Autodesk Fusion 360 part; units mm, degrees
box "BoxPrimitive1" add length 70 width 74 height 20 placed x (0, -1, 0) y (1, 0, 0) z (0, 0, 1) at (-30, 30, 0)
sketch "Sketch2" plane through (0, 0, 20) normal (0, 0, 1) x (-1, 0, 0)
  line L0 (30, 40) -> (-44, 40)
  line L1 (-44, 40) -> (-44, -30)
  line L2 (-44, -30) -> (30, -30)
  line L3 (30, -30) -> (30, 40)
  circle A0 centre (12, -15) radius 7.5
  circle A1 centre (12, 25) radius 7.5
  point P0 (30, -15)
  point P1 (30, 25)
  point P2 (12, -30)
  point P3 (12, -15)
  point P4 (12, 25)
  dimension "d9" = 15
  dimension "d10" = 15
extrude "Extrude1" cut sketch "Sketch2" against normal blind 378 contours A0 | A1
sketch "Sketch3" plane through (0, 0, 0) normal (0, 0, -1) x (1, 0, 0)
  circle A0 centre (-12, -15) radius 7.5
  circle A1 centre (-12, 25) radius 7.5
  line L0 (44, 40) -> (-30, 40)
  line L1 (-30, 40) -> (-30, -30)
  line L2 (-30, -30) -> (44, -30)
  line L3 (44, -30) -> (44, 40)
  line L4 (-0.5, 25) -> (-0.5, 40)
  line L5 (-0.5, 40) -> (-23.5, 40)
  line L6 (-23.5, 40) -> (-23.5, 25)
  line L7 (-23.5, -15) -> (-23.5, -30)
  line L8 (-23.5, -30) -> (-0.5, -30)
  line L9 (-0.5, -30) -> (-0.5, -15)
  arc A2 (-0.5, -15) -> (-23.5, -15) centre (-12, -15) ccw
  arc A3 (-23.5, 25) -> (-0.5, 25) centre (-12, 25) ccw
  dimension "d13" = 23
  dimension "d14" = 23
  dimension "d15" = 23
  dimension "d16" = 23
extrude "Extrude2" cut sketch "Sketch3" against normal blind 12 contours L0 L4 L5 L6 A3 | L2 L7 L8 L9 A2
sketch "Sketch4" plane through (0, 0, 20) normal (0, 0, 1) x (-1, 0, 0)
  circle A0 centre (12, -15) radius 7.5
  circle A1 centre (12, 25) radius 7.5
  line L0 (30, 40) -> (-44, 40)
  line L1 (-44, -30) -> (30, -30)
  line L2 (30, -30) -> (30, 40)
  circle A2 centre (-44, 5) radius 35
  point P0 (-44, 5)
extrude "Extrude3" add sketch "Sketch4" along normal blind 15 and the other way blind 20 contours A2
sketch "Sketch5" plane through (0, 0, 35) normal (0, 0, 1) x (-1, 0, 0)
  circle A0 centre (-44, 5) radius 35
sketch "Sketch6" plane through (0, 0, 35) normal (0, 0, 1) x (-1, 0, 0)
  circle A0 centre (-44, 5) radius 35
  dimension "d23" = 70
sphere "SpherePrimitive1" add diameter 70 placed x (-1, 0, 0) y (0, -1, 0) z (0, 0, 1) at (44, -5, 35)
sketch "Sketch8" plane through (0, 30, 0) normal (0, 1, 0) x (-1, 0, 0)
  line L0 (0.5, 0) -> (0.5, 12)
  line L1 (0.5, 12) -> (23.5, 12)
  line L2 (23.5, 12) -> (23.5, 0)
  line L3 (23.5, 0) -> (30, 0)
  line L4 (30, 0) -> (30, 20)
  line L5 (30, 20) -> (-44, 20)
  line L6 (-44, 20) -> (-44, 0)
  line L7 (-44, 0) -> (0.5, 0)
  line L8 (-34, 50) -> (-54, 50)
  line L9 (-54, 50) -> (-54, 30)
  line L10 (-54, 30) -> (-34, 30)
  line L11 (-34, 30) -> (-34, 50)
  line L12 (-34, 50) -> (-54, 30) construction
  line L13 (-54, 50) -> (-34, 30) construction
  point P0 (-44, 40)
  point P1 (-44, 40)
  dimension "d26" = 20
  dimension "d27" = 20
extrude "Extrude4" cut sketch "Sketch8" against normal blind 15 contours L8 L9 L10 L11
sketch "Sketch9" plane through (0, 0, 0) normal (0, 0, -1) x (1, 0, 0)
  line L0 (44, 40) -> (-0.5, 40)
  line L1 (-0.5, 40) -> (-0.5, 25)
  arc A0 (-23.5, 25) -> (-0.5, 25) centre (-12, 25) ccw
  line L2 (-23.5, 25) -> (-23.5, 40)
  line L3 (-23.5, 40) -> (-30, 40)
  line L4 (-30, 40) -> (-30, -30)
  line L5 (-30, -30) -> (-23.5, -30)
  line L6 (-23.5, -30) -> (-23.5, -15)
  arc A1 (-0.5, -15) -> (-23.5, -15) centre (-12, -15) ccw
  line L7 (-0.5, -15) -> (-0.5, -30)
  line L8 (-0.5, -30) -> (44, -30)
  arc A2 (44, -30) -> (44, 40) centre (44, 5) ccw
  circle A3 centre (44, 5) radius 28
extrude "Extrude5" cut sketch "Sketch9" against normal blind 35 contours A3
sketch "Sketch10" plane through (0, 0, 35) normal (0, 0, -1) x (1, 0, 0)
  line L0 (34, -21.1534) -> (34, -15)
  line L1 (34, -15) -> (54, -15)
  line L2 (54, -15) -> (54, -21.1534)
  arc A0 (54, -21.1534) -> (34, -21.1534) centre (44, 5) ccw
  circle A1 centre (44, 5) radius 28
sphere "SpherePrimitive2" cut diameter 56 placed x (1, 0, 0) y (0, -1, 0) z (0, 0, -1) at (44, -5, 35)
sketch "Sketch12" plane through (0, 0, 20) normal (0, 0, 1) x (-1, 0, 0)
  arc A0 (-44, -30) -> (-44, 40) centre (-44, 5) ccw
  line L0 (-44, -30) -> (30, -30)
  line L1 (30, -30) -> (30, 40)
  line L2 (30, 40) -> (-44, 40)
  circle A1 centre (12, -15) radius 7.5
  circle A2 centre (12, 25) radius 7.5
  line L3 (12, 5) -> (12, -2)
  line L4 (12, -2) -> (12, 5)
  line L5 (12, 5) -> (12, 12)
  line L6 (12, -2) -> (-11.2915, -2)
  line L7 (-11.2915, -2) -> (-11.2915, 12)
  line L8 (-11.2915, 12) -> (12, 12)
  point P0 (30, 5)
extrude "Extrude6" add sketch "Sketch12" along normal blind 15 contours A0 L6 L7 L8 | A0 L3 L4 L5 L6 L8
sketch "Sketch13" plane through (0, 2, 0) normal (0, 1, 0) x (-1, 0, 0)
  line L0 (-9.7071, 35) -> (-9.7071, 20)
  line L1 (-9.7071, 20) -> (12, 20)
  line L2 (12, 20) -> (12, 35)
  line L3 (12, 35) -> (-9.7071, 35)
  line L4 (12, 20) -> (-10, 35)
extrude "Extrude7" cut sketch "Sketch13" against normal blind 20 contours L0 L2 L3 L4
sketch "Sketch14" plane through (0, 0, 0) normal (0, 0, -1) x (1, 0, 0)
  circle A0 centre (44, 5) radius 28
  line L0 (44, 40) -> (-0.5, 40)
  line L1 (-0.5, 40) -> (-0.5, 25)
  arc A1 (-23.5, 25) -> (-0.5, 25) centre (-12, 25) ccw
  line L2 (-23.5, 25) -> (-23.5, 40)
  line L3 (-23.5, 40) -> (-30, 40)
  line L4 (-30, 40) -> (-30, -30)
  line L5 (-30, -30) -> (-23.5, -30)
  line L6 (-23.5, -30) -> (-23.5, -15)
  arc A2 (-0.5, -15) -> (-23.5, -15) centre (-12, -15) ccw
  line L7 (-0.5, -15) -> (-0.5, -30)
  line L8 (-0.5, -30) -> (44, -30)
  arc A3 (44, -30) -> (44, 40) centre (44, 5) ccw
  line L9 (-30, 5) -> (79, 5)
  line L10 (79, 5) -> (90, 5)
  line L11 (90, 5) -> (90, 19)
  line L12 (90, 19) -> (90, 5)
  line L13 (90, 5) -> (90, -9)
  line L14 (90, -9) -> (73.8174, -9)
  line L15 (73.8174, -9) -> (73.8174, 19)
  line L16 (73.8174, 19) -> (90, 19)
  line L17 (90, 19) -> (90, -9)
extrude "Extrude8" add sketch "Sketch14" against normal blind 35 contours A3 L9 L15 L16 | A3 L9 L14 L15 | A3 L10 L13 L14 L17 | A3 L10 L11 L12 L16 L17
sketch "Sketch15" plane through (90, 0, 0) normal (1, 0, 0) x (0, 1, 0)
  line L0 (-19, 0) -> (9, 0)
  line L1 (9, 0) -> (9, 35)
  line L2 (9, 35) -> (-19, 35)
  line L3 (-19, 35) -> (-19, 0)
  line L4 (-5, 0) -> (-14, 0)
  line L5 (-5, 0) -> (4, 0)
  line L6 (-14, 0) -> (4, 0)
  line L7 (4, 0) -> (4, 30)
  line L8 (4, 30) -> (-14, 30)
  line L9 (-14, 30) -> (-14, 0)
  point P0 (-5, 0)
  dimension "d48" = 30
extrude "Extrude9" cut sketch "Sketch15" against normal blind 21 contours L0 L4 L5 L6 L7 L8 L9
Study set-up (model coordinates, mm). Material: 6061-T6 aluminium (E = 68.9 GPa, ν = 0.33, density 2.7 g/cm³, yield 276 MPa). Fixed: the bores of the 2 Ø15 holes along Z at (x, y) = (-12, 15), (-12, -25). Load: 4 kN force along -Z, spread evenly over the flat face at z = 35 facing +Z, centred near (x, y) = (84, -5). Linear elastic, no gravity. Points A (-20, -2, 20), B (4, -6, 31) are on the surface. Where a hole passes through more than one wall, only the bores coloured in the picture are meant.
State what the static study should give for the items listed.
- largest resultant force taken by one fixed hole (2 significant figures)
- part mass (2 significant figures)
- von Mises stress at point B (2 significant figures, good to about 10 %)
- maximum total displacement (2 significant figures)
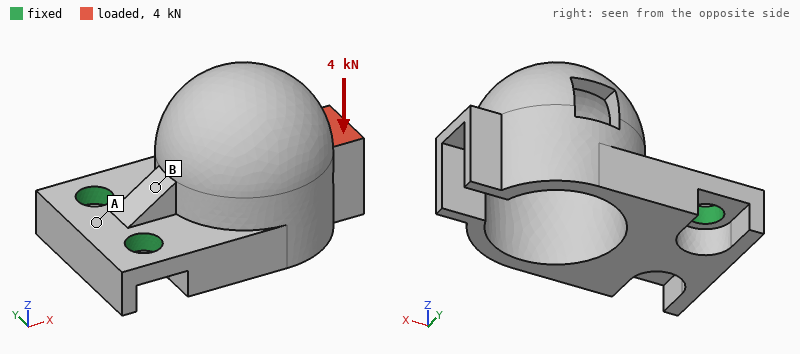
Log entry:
3.5 kN
380 g
95 MPa
0.85 mm
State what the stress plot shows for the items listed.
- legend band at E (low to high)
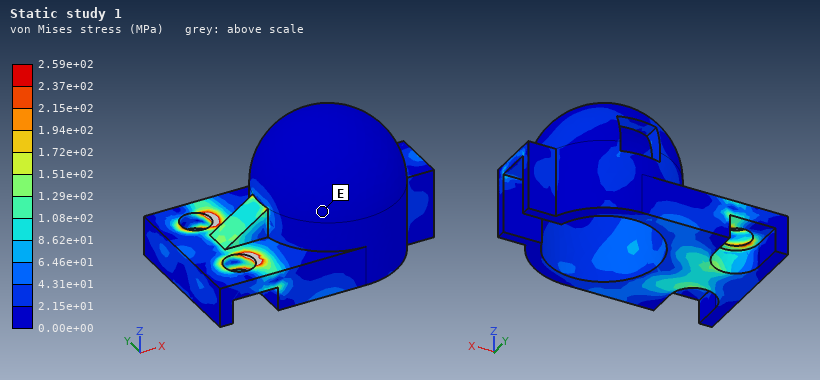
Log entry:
0.00e+00 to 2.15e+01 MPa
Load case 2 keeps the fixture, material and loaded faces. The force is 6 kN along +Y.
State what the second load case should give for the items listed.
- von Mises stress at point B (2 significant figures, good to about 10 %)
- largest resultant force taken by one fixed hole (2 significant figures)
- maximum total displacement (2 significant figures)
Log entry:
28 MPa
12 kN
0.44 mm
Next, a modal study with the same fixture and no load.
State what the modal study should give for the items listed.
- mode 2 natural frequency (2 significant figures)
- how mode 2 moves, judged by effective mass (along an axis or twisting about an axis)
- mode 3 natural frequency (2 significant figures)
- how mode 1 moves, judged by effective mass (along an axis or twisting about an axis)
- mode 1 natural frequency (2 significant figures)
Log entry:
2000 Hz
along Y
3000 Hz
along Z
1100 Hz
